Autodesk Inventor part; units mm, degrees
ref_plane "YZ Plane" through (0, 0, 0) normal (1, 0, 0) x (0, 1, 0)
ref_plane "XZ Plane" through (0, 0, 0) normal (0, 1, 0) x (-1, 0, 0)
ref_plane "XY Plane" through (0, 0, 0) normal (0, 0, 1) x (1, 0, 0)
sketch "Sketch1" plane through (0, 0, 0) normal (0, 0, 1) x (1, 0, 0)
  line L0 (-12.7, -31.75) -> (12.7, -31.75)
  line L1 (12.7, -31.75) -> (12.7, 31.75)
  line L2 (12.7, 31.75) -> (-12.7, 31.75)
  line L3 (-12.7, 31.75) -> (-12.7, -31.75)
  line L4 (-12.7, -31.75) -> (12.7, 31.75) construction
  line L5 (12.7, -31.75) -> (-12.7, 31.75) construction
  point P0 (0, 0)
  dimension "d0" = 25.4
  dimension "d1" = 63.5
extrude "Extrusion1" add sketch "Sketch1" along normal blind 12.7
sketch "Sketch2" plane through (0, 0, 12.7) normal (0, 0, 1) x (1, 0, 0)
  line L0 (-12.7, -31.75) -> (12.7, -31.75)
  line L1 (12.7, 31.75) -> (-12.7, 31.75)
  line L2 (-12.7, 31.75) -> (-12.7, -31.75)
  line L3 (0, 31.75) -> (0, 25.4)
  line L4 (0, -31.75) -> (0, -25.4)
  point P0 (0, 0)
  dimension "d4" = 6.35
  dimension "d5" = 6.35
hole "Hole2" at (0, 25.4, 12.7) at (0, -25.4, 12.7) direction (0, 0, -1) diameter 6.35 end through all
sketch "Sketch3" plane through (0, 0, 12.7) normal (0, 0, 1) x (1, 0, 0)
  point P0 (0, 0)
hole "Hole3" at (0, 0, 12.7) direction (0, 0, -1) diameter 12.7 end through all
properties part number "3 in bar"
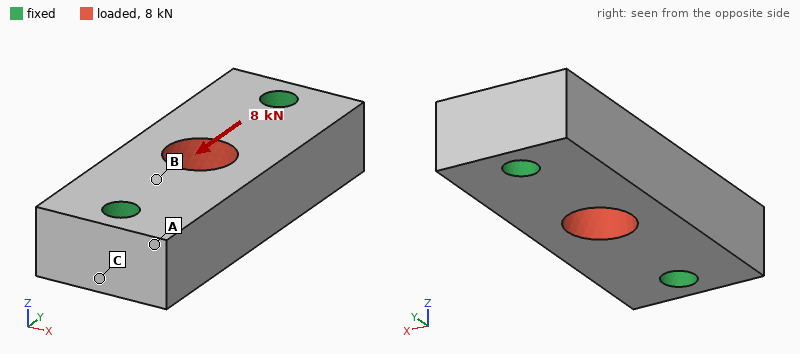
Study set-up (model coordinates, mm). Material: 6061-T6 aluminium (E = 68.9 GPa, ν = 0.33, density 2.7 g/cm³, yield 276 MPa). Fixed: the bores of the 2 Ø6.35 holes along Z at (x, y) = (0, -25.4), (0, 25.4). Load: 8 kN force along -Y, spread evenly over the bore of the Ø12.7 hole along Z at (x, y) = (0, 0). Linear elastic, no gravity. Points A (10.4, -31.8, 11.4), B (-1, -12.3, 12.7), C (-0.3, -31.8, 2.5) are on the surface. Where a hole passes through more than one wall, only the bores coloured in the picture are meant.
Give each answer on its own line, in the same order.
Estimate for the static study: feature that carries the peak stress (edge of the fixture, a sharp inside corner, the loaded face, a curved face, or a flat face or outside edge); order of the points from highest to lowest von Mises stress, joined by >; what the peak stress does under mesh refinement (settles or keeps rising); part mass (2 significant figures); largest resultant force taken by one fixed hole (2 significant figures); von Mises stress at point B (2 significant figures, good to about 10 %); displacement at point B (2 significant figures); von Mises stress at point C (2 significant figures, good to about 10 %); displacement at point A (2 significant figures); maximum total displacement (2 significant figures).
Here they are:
edge of the fixture
B > C > A
keeps rising
49 g
4.0 kN
20 MPa
3.3 µm
13 MPa
2.4 µm
5.9 µm
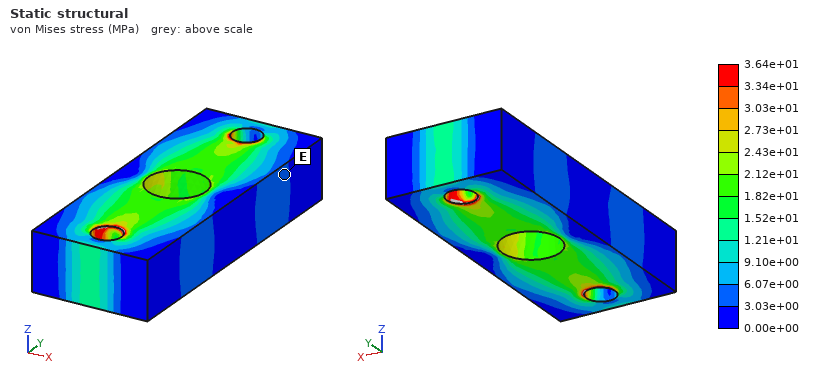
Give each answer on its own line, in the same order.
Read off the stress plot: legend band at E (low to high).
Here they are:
3.03e+00 to 6.07e+00 MPa
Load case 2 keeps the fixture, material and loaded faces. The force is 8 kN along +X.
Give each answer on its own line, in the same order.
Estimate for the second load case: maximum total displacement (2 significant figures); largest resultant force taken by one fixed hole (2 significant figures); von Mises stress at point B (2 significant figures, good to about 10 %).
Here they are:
23 µm
4.0 kN
31 MPa
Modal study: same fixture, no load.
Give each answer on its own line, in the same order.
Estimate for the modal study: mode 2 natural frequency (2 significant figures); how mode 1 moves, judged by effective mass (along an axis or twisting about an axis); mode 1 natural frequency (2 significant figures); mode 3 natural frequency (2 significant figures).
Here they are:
22 kHz
along Z
19 kHz
23 kHz
